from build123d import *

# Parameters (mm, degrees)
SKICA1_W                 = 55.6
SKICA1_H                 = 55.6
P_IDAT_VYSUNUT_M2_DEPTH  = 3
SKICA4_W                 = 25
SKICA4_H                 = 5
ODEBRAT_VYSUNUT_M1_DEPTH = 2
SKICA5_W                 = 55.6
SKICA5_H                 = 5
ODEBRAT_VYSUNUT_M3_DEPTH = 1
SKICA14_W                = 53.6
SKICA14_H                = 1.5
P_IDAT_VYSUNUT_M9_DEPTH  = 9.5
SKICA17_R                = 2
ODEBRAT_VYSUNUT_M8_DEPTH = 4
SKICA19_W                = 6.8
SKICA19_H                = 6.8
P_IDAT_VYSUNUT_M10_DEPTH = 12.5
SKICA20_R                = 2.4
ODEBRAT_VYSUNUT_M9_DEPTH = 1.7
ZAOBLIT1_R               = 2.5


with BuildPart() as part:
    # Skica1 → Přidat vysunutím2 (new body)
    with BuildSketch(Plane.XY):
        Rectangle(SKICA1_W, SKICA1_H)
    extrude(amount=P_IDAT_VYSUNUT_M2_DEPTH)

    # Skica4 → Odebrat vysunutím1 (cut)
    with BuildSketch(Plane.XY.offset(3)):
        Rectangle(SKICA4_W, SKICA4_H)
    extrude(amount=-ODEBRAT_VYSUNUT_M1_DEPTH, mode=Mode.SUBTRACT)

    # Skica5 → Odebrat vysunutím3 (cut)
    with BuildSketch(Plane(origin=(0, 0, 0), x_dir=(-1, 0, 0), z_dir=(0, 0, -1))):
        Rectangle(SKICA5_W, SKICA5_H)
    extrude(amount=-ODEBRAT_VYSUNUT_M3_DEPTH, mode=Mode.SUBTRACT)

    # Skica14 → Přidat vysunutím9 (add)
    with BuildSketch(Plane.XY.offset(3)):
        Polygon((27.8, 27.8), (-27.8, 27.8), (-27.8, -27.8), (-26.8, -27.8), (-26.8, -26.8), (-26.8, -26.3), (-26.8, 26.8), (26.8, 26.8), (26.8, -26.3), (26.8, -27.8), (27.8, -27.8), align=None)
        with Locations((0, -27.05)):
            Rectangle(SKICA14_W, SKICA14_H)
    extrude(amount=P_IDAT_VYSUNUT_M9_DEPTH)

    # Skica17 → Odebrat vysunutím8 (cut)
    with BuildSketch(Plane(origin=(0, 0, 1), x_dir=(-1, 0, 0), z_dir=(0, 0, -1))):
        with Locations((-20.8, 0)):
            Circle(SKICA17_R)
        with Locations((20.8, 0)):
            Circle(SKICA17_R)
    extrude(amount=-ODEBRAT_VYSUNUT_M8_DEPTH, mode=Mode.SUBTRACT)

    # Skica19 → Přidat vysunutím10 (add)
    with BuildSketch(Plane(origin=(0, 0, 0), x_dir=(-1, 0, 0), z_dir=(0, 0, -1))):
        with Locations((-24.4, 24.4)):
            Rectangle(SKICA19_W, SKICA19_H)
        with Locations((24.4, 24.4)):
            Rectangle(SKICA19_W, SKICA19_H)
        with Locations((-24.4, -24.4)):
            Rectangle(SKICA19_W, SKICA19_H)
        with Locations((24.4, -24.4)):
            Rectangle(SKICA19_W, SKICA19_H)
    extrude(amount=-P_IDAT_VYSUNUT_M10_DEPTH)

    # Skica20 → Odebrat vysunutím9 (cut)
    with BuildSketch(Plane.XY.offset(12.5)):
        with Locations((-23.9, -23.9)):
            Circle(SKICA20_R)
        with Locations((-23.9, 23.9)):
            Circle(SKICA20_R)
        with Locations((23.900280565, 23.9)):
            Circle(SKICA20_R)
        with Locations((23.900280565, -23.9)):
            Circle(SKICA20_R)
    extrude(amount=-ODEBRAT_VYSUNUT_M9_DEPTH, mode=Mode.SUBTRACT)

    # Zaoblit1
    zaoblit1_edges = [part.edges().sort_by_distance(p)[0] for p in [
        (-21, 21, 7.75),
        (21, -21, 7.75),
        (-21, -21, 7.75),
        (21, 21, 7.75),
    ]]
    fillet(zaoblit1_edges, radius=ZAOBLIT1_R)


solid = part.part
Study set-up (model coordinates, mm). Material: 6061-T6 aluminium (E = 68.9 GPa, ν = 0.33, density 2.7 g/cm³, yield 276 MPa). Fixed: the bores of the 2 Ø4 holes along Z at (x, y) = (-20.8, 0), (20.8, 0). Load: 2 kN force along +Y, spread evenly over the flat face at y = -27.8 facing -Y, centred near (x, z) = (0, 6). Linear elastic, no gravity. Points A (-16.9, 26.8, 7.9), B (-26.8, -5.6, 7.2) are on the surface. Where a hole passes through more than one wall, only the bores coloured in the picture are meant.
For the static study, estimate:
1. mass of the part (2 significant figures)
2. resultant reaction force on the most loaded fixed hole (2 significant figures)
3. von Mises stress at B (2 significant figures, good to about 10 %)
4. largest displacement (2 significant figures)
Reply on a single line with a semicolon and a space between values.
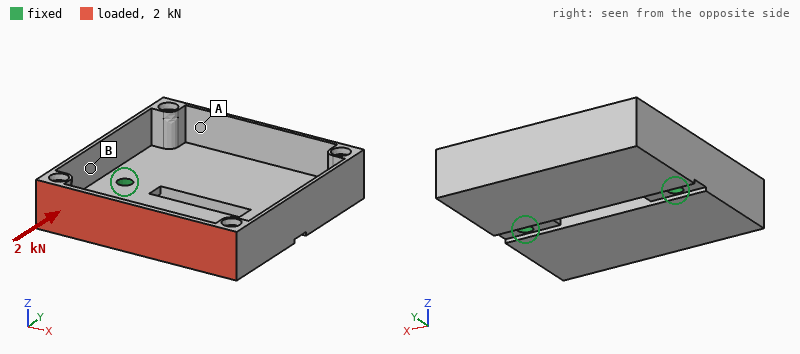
33 g; 1.0 kN; 44 MPa; 0.41 mm
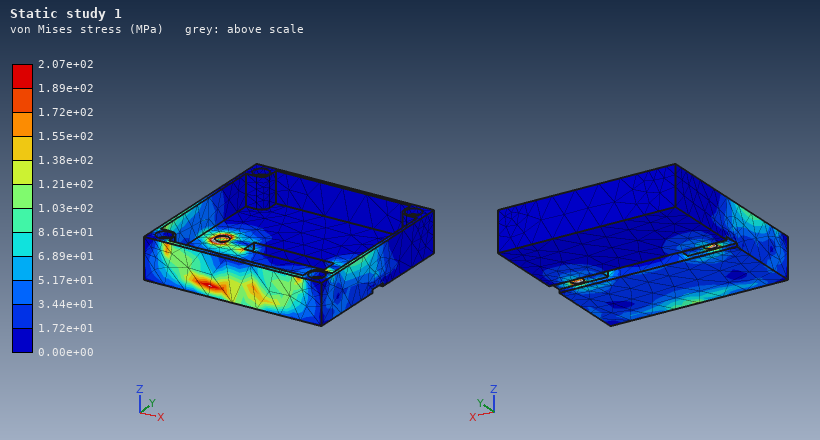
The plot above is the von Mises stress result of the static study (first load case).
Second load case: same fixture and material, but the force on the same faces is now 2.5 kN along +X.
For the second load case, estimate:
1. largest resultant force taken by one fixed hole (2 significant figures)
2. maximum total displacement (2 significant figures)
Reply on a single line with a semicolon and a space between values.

2.0 kN; 0.30 mm
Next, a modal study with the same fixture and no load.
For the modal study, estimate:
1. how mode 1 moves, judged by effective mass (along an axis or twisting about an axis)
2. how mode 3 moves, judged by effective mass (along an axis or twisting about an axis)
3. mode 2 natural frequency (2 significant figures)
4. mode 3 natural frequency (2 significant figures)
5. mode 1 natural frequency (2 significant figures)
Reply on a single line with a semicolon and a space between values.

twisting about X; along Z; 2900 Hz; 3700 Hz; 1700 Hz
